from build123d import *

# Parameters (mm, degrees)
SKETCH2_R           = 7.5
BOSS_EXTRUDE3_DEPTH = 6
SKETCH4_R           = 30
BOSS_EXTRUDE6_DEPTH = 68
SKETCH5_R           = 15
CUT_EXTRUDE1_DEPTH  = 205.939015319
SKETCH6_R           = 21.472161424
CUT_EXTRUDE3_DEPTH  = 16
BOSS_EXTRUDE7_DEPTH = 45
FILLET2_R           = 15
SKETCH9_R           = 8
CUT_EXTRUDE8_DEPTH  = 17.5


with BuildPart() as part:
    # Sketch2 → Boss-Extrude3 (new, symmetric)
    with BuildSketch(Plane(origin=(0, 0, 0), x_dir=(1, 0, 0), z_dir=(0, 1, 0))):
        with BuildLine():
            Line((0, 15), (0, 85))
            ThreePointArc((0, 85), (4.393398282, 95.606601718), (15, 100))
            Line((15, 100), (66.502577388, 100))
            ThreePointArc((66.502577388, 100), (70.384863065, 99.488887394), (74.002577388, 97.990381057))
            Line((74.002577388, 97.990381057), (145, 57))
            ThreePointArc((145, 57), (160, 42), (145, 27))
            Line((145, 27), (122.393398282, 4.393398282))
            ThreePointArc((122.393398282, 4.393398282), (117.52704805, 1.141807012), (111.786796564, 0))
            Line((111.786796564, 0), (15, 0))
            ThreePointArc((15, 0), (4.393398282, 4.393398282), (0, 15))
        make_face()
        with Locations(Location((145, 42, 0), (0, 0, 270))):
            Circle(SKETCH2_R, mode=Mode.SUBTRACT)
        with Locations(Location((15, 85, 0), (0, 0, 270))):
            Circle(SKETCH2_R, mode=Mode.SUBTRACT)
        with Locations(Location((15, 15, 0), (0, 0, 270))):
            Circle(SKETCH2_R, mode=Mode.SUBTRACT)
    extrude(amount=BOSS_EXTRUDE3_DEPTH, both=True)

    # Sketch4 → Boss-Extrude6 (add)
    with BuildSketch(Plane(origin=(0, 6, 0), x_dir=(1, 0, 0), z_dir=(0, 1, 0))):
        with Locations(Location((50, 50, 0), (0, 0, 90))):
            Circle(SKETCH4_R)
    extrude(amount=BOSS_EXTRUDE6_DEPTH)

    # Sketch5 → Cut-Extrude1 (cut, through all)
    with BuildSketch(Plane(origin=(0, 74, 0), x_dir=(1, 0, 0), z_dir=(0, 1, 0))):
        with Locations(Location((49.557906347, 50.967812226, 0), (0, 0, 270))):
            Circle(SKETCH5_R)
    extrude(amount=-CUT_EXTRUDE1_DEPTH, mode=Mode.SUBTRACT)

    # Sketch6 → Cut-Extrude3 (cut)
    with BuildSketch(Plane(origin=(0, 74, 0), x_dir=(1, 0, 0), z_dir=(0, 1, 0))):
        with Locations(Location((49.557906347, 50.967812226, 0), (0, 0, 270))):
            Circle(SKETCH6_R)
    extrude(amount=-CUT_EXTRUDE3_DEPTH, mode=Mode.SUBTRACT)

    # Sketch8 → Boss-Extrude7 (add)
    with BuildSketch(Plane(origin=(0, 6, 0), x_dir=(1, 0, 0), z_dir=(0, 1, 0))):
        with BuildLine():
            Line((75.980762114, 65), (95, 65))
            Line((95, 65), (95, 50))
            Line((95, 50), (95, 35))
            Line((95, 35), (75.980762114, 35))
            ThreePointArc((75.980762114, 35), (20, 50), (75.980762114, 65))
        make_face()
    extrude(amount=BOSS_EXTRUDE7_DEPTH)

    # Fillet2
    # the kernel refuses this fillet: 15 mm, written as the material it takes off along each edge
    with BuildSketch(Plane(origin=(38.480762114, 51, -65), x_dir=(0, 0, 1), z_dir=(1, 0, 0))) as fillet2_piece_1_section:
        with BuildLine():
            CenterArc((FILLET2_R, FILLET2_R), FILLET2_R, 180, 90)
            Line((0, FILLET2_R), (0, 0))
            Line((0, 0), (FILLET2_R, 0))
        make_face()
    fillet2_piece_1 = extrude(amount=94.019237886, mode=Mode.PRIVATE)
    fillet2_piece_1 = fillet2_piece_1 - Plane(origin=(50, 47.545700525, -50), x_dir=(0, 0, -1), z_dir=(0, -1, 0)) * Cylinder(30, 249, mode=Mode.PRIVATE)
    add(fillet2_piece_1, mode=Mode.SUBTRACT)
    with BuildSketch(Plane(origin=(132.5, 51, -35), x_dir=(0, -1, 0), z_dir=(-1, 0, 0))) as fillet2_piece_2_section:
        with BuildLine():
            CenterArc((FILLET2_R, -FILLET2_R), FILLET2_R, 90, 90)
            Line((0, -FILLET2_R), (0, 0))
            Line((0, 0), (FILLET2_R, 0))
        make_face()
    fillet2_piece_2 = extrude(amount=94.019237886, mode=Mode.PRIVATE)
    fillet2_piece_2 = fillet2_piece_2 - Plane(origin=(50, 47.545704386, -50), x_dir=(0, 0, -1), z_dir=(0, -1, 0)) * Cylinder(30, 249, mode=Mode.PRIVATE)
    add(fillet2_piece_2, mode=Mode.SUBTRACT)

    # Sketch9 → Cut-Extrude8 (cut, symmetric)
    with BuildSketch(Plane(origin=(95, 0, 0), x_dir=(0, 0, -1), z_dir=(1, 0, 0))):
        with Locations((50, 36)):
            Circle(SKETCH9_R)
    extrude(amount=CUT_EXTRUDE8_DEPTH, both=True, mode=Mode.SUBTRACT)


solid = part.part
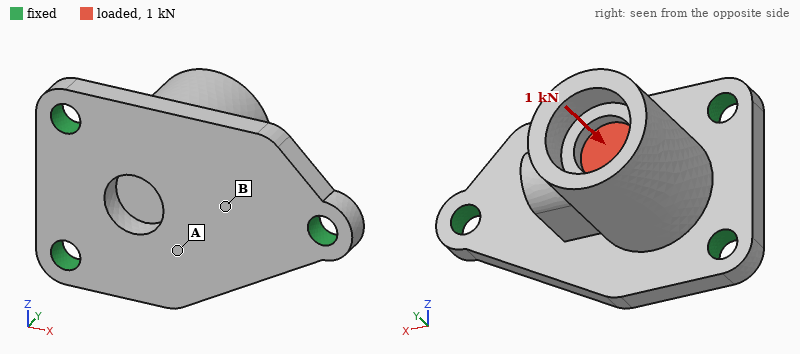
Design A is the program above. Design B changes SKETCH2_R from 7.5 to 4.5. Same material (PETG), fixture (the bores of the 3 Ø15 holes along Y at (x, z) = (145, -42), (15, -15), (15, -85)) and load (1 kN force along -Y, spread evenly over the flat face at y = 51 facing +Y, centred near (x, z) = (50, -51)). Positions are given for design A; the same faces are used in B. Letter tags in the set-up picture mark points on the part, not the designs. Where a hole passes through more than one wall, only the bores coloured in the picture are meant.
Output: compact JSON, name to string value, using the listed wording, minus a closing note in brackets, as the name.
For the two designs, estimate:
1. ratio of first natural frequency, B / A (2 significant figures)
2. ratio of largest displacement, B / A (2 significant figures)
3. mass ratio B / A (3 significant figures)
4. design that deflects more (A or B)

{"ratio of first natural frequency, B / A": "0.90", "ratio of largest displacement, B / A": "1.3", "mass ratio B / A": "1.01", "design that deflects more": "B"}
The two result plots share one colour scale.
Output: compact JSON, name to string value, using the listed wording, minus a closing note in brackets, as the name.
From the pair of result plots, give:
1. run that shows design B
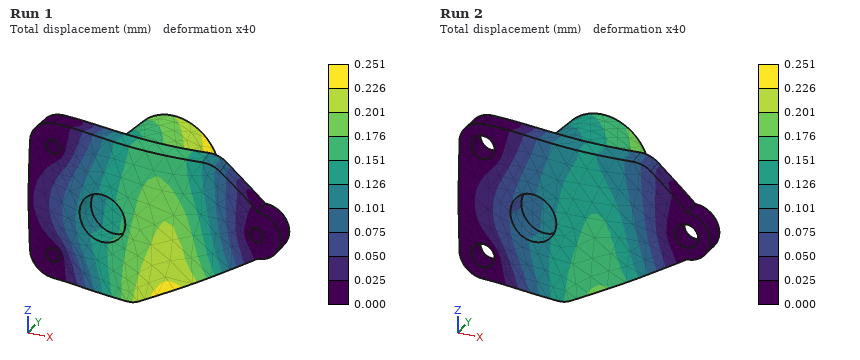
{"run that shows design B": "Run 1"}
